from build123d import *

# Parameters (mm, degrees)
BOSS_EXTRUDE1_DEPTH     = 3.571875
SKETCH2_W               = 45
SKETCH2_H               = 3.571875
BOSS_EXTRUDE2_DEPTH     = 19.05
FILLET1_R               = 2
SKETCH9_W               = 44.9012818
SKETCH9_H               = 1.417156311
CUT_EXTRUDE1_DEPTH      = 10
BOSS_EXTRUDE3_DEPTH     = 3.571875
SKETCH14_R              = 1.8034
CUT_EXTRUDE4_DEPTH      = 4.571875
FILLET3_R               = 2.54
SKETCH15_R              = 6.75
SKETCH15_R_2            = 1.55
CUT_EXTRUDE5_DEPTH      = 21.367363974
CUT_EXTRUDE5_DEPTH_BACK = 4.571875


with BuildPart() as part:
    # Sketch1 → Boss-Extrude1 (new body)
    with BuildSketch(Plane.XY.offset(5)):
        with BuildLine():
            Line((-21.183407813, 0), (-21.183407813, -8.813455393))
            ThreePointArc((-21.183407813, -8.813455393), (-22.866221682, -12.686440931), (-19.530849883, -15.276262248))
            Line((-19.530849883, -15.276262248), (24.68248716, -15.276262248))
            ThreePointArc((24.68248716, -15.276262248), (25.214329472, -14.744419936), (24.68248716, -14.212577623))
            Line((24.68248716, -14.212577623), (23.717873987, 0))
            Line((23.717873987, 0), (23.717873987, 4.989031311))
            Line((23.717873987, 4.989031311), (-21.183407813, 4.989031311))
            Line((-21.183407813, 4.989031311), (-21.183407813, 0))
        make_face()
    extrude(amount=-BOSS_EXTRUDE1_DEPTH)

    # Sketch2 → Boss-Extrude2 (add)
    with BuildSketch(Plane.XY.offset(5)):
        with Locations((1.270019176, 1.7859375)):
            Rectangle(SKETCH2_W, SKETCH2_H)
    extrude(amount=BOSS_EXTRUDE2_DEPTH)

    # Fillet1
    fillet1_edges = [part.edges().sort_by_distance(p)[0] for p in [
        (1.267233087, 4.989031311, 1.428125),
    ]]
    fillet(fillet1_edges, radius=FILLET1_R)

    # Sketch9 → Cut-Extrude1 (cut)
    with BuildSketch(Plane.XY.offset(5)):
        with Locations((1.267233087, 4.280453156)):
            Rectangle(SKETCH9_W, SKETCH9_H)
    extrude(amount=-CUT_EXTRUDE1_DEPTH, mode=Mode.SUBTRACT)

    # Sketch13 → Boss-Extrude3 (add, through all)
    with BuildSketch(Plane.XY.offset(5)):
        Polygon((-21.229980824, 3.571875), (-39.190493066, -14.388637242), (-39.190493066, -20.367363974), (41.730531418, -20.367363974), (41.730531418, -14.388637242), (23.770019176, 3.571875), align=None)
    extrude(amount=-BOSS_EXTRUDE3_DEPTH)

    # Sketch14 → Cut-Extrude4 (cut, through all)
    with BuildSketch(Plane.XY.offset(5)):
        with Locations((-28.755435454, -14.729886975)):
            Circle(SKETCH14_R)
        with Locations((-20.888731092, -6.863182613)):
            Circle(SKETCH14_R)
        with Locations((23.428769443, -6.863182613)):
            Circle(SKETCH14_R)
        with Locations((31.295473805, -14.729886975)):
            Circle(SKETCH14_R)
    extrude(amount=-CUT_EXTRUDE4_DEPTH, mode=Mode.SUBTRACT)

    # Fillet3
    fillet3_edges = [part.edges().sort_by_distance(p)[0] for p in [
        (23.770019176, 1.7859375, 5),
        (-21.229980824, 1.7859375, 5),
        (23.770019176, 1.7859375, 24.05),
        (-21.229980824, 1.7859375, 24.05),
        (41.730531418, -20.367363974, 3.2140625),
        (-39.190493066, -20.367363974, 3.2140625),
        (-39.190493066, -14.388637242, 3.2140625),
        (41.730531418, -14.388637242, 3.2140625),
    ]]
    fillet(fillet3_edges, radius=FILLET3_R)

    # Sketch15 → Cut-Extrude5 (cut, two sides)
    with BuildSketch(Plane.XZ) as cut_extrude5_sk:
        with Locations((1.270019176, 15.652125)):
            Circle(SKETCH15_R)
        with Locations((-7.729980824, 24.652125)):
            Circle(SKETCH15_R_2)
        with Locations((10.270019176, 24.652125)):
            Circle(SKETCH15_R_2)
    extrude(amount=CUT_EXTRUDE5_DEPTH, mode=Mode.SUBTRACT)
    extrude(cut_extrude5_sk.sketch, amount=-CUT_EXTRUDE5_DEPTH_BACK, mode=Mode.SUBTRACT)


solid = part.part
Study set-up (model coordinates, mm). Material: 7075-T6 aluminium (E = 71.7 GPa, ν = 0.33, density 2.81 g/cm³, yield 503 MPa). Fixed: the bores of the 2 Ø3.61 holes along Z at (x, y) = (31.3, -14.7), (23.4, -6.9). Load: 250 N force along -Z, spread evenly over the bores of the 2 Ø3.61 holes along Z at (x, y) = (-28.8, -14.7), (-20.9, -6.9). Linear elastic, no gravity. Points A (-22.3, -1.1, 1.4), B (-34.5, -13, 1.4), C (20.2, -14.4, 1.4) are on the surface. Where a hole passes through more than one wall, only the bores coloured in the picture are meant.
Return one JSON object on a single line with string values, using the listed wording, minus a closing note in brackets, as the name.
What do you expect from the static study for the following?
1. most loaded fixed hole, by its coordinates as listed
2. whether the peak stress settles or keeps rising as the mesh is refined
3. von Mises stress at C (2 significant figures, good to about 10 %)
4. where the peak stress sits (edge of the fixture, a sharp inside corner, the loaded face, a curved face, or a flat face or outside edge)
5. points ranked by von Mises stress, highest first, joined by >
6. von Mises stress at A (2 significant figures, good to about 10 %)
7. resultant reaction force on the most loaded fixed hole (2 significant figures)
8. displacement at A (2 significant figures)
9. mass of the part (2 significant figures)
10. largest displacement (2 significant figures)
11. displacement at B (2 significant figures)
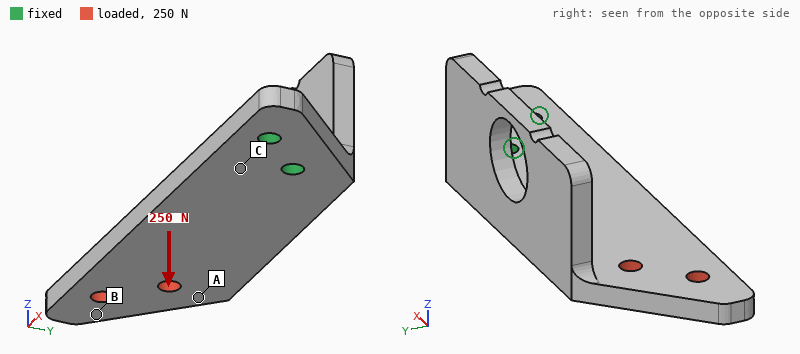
{"most loaded fixed hole, by its coordinates as listed": "(23.4, -6.9)", "whether the peak stress settles or keeps rising as the mesh is refined": "keeps rising", "von Mises stress at C": "110 MPa", "where the peak stress sits": "edge of the fixture", "points ranked by von Mises stress, highest first, joined by >": "C > A > B", "von Mises stress at A": "61 MPa", "resultant reaction force on the most loaded fixed hole": "530 N", "displacement at A": "0.56 mm", "mass of the part": "23 g", "largest displacement": "0.95 mm", "displacement at B": "0.84 mm"}
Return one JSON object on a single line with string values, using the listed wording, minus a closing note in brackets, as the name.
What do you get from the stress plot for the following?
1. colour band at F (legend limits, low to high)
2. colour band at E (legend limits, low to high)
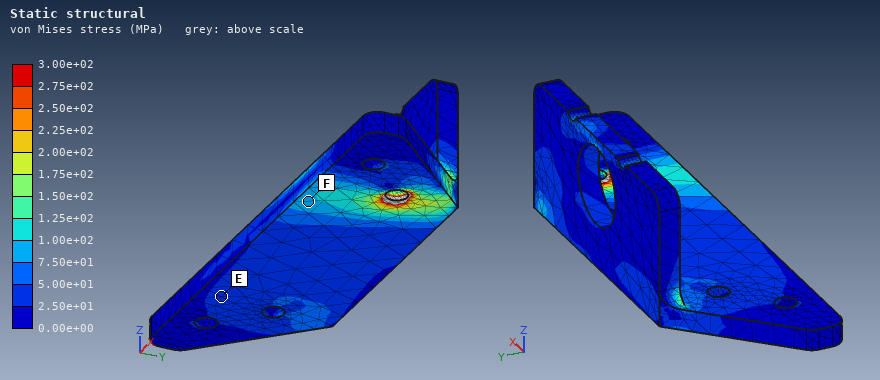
{"colour band at F": "7.50e+01 to 1.00e+02 MPa", "colour band at E": "2.50e+01 to 5.00e+01 MPa"}
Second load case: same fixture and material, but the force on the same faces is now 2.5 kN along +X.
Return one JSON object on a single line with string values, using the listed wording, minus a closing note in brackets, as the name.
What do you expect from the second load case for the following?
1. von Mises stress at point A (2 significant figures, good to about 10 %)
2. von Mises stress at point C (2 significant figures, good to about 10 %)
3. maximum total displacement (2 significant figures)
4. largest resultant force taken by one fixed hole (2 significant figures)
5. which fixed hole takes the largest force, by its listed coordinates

{"von Mises stress at point A": "11 MPa", "von Mises stress at point C": "34 MPa", "maximum total displacement": "63 µm", "largest resultant force taken by one fixed hole": "1.4 kN", "which fixed hole takes the largest force, by its listed coordinates": "(23.4, -6.9)"}
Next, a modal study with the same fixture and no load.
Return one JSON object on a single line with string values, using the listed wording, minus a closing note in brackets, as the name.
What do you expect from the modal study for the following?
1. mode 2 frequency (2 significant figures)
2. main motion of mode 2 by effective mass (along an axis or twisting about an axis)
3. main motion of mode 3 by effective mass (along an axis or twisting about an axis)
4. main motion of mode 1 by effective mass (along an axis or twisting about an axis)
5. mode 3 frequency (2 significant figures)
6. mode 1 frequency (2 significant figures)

{"mode 2 frequency": "2400 Hz", "main motion of mode 2 by effective mass": "along Y", "main motion of mode 3 by effective mass": "along Y", "main motion of mode 1 by effective mass": "along Z", "mode 3 frequency": "3800 Hz", "mode 1 frequency": "1100 Hz"}
